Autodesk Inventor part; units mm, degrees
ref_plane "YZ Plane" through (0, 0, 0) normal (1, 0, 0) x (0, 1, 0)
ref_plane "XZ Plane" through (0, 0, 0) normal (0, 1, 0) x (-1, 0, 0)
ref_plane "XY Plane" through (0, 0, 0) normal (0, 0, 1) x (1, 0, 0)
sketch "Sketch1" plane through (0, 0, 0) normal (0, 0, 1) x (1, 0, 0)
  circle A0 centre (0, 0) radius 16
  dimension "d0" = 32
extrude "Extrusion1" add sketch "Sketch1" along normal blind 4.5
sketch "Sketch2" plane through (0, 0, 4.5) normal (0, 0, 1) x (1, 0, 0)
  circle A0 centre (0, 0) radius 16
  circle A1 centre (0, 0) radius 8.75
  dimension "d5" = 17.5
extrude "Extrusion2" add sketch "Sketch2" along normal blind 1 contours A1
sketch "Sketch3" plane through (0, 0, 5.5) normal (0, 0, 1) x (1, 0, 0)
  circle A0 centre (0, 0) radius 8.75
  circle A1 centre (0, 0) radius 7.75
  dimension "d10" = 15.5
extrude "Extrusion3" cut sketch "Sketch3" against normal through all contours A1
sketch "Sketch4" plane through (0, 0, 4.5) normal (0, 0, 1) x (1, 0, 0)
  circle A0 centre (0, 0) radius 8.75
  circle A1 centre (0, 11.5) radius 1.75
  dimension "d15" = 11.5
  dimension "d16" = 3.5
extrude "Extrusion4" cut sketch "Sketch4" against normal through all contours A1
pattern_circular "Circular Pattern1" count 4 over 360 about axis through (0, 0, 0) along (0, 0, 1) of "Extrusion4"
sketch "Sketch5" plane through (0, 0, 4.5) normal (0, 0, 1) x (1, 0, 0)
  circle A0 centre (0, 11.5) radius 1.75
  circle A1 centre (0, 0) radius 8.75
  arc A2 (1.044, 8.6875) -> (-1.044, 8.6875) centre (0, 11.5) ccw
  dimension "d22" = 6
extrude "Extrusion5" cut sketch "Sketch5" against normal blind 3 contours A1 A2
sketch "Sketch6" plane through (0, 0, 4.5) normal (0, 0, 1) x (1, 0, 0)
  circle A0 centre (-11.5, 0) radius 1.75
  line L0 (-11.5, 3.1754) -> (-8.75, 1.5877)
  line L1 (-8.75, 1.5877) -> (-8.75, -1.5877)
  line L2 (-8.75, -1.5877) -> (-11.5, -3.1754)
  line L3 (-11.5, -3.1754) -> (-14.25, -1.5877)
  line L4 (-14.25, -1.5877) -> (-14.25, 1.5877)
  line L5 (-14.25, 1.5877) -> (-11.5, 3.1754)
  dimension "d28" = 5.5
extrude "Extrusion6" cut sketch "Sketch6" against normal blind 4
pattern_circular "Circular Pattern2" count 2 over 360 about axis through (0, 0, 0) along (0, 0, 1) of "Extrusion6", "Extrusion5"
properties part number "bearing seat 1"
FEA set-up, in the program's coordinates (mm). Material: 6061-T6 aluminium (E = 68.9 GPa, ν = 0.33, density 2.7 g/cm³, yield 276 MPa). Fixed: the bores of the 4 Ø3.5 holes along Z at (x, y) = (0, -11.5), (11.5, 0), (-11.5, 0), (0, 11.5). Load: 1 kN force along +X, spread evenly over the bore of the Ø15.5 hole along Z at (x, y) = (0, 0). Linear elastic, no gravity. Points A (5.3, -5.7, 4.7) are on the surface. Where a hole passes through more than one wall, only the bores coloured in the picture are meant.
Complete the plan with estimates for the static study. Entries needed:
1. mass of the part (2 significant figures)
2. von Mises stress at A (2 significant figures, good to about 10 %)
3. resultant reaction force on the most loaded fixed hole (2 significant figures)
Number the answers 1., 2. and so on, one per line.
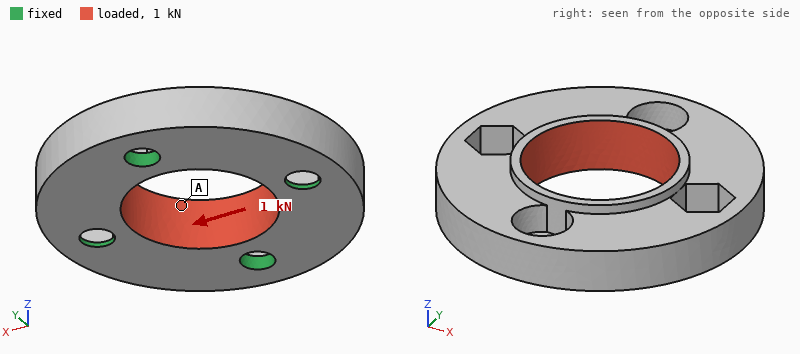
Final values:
1. 6.5 g
2. 10 MPa
3. 350 N
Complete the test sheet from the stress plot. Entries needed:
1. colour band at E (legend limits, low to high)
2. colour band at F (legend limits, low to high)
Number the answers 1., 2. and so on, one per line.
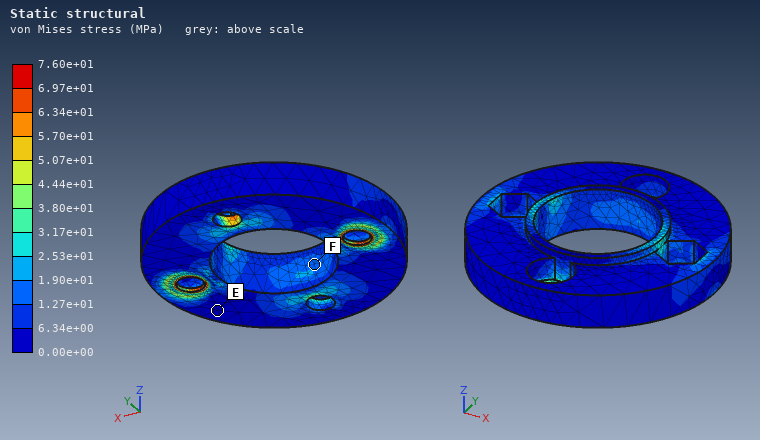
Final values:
1. 0.00e+00 to 6.34e+00 MPa
2. 1.27e+01 to 1.90e+01 MPa
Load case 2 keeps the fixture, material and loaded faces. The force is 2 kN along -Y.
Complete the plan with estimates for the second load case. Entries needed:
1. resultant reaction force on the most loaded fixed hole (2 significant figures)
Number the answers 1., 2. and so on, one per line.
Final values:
1. 620 N
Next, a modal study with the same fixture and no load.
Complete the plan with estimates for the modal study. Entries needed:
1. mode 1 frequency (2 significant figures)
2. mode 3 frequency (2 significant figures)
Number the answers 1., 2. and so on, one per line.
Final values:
1. 20 kHz
2. 26 kHz
